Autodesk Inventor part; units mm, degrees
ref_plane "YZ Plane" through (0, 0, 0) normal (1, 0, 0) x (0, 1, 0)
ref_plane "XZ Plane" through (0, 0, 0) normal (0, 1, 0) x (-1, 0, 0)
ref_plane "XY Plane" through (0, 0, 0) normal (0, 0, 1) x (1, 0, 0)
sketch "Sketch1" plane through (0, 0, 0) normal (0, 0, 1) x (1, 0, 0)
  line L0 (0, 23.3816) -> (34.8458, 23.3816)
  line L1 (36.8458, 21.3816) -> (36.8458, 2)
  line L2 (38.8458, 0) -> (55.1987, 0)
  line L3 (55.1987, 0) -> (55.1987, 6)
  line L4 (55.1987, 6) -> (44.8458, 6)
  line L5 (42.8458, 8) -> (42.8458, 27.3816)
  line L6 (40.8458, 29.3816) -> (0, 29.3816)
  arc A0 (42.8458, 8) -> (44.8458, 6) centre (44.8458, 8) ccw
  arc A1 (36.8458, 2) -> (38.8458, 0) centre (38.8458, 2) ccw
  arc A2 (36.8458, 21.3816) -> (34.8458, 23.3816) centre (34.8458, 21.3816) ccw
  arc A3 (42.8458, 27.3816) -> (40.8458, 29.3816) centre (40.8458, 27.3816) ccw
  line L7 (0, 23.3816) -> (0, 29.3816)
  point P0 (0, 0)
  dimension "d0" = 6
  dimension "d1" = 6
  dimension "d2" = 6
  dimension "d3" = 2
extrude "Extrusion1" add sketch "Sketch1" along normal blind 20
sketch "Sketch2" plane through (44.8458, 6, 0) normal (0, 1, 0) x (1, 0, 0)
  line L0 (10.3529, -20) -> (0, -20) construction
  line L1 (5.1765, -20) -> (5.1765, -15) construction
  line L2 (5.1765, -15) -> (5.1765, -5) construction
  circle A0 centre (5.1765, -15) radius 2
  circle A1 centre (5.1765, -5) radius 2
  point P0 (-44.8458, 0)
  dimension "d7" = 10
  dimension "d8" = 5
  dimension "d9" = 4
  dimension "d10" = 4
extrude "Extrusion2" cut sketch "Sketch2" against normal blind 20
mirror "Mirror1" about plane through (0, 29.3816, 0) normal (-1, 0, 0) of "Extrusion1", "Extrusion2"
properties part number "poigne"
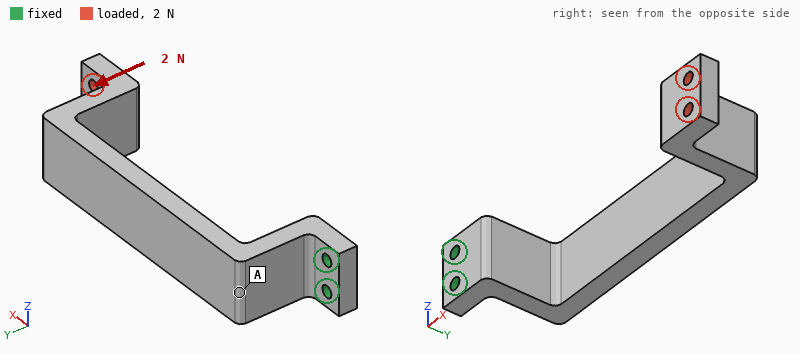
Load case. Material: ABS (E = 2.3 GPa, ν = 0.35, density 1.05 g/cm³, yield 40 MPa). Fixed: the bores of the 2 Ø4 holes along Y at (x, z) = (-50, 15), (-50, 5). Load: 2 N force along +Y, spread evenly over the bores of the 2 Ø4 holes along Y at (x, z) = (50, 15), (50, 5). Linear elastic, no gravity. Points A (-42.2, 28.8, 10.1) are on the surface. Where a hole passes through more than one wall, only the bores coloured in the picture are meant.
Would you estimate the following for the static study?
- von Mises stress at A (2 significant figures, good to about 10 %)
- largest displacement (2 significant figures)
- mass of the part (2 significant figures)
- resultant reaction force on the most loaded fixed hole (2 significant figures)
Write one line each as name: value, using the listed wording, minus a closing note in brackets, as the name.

von Mises stress at A: 0.26 MPa
largest displacement: 1.2 mm
mass of the part: 19 g
resultant reaction force on the most loaded fixed hole: 2.2 N
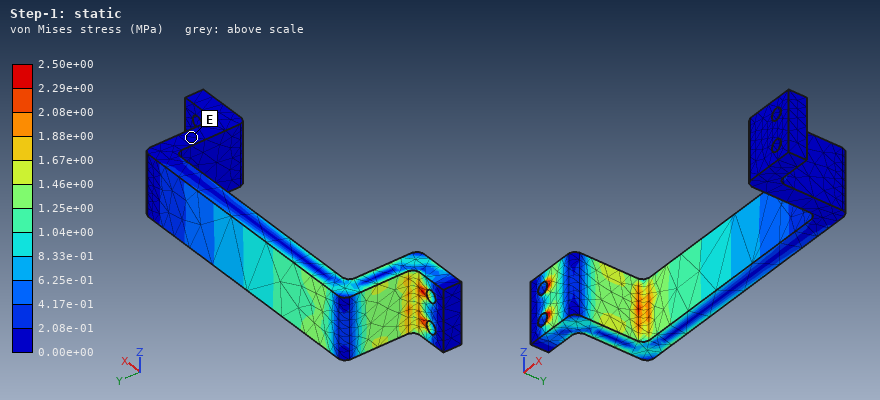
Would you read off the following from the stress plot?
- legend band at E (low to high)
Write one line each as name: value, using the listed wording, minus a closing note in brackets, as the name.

legend band at E: 0.00e+00 to 2.08e-01 MPa
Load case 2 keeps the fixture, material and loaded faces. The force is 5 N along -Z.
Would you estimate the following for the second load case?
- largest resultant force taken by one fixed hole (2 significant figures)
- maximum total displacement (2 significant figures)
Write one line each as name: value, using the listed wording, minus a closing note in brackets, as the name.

largest resultant force taken by one fixed hole: 40 N
maximum total displacement: 1.2 mm
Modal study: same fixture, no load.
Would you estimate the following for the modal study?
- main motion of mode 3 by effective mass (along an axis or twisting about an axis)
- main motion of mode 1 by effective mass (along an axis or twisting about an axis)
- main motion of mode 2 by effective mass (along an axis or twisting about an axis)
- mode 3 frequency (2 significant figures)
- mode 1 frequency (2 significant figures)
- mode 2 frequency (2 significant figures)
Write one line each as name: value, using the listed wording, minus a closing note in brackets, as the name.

main motion of mode 3 by effective mass: along X
main motion of mode 1 by effective mass: along Y
main motion of mode 2 by effective mass: along Z
mode 3 frequency: 390 Hz
mode 1 frequency: 87 Hz
mode 2 frequency: 150 Hz
